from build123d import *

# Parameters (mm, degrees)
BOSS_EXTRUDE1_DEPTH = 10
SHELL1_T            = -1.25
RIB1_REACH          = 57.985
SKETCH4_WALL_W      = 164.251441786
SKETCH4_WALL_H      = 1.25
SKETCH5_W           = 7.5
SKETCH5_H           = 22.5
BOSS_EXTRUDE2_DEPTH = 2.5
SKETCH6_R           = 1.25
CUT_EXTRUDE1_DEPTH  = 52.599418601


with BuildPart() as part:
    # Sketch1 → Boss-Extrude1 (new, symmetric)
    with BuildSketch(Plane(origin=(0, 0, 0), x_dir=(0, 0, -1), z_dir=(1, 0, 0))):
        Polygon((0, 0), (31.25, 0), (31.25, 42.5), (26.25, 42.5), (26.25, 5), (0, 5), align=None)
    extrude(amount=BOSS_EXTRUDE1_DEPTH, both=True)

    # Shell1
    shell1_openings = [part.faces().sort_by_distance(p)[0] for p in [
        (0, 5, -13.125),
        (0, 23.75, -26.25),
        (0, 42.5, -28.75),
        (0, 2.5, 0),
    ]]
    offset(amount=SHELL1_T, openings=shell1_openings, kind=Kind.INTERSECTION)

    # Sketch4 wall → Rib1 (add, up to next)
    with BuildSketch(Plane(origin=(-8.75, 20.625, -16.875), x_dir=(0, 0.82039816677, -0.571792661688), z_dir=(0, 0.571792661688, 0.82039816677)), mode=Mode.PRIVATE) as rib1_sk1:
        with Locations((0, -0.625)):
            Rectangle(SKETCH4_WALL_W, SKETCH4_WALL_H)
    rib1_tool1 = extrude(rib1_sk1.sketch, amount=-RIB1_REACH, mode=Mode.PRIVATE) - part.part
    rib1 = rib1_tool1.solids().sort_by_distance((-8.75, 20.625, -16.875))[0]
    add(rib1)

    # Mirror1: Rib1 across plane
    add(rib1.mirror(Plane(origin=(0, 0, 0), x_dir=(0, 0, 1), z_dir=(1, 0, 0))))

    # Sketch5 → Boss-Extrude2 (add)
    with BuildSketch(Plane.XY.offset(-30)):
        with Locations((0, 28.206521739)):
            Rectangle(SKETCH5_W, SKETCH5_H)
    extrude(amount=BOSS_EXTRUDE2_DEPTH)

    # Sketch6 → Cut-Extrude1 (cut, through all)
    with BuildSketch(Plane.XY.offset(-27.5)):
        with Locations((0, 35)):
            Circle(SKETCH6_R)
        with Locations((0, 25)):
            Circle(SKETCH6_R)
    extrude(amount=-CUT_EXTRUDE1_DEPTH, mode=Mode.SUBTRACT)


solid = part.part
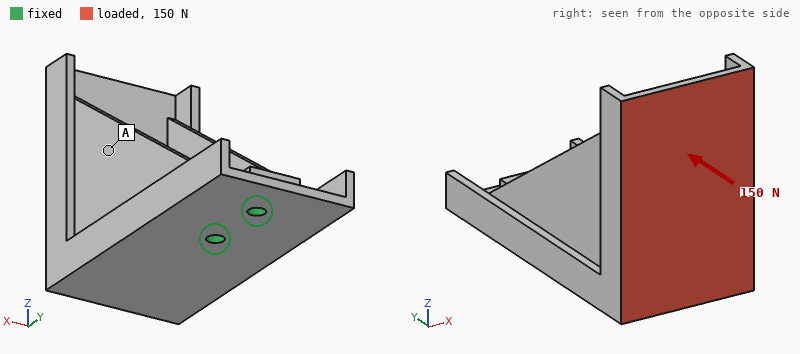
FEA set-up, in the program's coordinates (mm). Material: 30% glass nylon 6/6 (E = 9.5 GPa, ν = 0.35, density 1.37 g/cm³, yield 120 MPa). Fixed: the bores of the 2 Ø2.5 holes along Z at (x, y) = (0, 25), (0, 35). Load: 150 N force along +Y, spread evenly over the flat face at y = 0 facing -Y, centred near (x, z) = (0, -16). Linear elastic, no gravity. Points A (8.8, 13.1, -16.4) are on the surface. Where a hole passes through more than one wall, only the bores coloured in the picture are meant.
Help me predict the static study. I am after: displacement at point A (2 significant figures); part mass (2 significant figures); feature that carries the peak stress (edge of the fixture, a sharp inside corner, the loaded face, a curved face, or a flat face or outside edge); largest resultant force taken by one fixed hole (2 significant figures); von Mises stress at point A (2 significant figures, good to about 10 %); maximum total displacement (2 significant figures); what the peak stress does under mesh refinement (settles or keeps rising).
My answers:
0.25 mm
5.6 g
edge of the fixture
150 N
6.2 MPa
0.65 mm
keeps rising
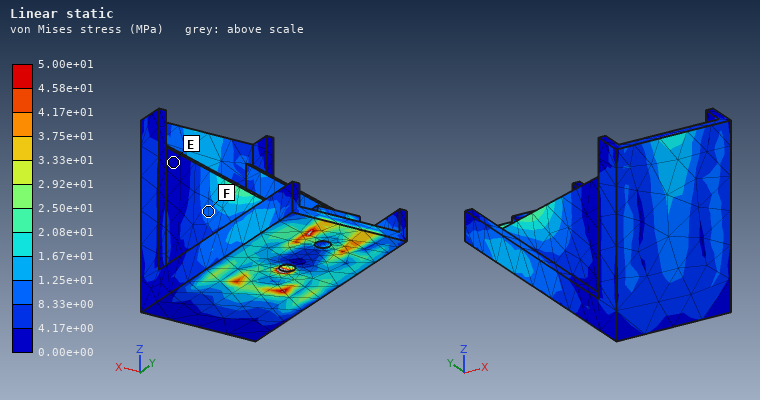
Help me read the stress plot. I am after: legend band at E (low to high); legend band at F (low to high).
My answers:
0.00e+00 to 4.17e+00 MPa
8.33e+00 to 1.25e+01 MPa
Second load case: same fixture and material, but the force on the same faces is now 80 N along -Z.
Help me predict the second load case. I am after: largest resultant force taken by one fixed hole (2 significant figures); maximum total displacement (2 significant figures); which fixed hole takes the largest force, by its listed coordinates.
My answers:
180 N
0.57 mm
(0, 25)
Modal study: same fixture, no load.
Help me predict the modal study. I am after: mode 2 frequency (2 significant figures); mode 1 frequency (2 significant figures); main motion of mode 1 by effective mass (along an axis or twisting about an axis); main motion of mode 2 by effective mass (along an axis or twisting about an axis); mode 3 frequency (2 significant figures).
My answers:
1300 Hz
770 Hz
along X
along Z
3400 Hz
